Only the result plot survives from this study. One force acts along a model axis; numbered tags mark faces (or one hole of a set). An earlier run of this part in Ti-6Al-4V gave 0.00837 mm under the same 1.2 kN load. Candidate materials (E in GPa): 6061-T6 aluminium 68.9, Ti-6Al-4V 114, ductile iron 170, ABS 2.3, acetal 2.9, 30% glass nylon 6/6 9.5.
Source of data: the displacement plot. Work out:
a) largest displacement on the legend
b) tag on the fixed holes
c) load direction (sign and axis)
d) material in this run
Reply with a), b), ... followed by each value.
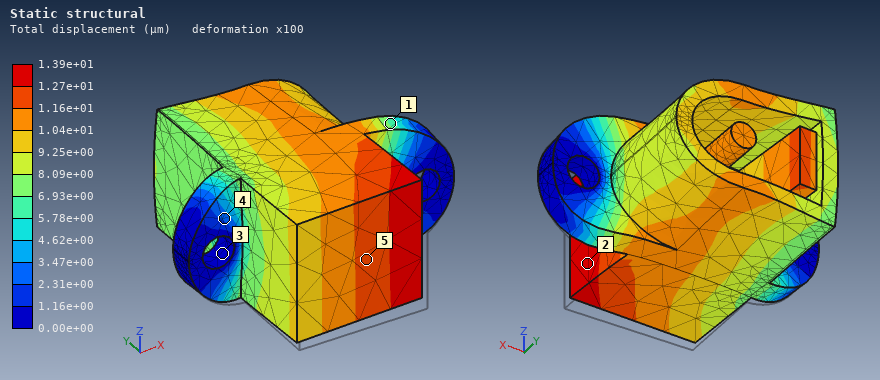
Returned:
a) 1.39e+01 µm
b) 3
c) +Y
d) 6061-T6 aluminium
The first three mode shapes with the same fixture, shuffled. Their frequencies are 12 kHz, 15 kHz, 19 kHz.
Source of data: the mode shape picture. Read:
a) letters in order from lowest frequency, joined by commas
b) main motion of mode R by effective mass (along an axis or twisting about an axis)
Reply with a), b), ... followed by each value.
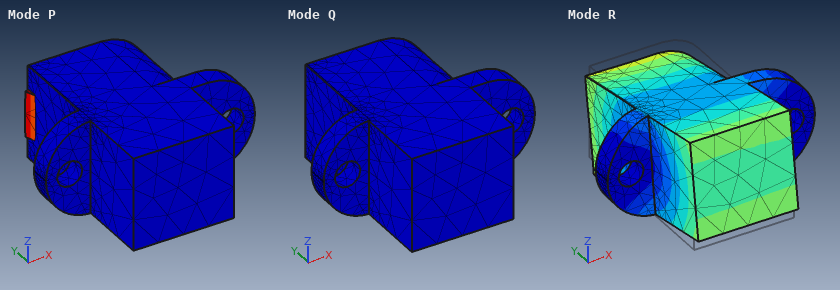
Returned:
a) R, P, Q
b) twisting about X
